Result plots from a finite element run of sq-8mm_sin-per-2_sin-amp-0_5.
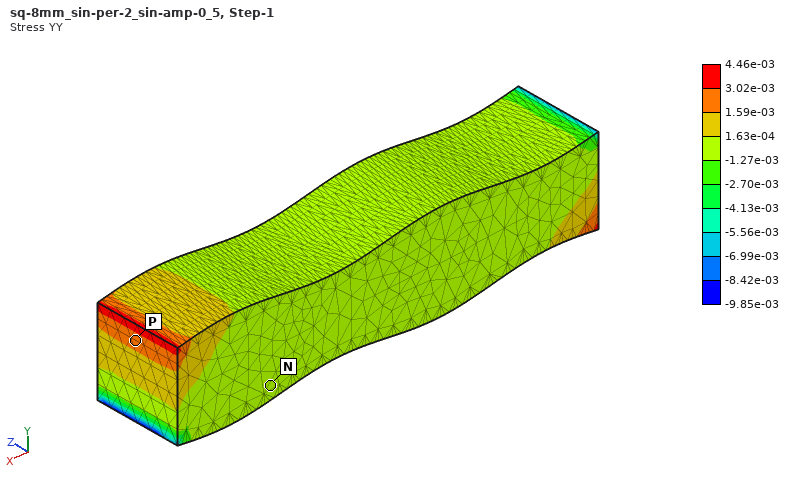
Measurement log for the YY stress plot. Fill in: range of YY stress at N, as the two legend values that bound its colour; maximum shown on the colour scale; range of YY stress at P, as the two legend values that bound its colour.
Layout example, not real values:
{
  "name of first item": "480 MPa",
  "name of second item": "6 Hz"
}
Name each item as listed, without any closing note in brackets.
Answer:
{
  "range of YY stress at N, as the two legend values that bound its colour": "-1.27e-03 to 1.63e-04",
  "maximum shown on the colour scale": "4.46e-03",
  "range of YY stress at P, as the two legend values that bound its colour": "1.59e-03 to 3.02e-03"
}
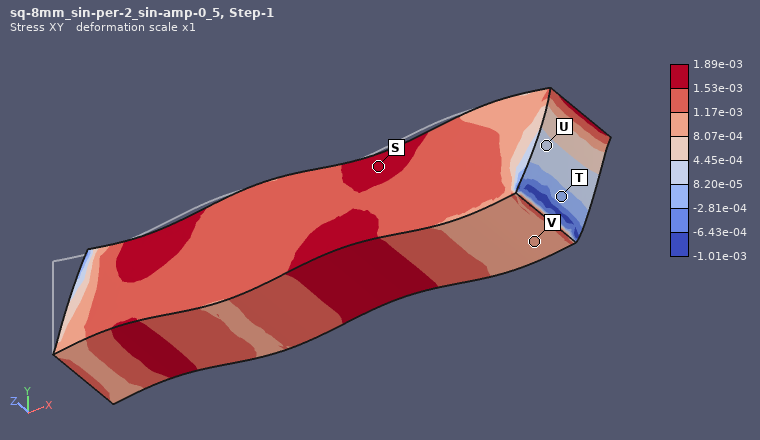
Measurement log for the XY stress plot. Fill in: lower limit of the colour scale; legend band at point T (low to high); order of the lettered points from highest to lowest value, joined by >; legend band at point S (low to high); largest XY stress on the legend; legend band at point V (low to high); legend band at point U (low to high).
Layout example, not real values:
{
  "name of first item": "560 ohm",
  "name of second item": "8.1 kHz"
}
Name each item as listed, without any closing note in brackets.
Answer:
{
  "lower limit of the colour scale": "-1.01e-03",
  "legend band at point T": "-2.81e-04 to 8.20e-05",
  "order of the lettered points from highest to lowest value, joined by >": "S > V > U > T",
  "legend band at point S": "1.53e-03 to 1.89e-03",
  "largest XY stress on the legend": "1.89e-03",
  "legend band at point V": "8.07e-04 to 1.17e-03",
  "legend band at point U": "8.20e-05 to 4.45e-04"
}
